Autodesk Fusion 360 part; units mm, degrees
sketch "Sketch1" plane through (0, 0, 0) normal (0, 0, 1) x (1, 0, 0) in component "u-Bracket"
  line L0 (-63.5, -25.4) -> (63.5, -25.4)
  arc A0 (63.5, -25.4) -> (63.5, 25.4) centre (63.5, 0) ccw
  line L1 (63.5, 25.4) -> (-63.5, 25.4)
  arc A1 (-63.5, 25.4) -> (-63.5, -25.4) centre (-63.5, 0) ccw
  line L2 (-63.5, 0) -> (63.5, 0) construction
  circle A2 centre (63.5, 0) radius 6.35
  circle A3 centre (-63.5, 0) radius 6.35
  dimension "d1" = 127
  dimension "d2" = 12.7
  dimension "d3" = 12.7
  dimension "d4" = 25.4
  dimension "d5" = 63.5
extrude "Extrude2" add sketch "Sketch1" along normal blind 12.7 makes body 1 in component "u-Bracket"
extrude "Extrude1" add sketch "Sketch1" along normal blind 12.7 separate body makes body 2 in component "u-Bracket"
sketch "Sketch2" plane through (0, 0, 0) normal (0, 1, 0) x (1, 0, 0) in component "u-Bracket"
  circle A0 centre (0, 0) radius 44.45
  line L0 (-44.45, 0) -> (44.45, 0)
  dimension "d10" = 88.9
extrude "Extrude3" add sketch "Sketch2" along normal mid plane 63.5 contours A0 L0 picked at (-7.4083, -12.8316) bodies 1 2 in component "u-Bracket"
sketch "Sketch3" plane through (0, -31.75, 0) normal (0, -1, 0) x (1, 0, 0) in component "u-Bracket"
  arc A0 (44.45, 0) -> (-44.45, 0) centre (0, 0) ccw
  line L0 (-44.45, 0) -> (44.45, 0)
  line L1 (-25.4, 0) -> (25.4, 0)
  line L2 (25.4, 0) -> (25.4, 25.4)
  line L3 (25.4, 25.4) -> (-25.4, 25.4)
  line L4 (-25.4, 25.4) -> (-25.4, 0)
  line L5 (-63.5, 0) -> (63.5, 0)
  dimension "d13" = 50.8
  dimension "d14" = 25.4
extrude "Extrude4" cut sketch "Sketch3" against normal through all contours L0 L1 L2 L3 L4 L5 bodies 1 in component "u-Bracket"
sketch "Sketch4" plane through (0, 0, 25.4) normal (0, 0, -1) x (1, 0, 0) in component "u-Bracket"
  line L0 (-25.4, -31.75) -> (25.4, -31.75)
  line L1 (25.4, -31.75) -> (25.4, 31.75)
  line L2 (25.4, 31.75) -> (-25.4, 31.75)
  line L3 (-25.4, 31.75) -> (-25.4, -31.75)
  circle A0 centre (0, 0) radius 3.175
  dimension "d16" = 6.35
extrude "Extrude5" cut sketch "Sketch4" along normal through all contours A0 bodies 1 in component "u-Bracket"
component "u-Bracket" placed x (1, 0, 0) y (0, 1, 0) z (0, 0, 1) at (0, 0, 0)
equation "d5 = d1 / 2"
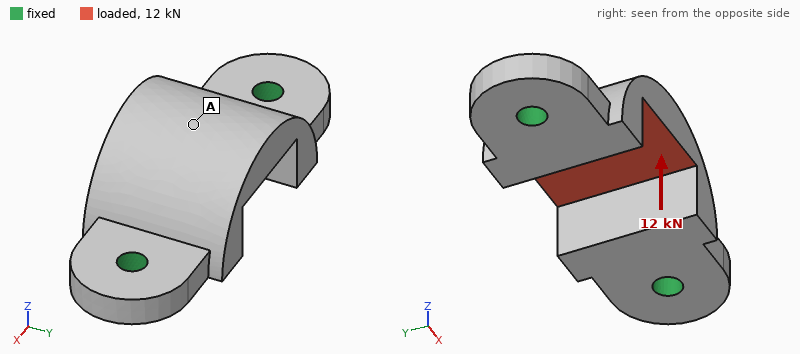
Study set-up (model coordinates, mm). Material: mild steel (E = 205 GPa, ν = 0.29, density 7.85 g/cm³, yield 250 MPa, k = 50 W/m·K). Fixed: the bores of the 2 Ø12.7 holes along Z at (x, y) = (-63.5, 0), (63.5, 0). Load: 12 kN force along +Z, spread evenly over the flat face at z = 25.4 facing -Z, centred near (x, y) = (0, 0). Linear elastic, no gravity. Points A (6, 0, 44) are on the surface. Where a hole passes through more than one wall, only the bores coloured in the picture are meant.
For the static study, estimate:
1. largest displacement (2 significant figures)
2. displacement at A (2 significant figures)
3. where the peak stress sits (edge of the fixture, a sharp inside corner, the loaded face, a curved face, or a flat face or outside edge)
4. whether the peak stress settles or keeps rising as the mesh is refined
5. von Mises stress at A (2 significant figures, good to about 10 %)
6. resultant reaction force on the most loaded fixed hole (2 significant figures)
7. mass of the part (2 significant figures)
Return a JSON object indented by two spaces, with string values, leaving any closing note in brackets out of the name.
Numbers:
{
  "largest displacement": "15 µm",
  "displacement at A": "14 µm",
  "where the peak stress sits": "edge of the fixture",
  "whether the peak stress settles or keeps rising as the mesh is refined": "keeps rising",
  "von Mises stress at A": "14 MPa",
  "resultant reaction force on the most loaded fixed hole": "8.6 kN",
  "mass of the part": "1.3 kg"
}
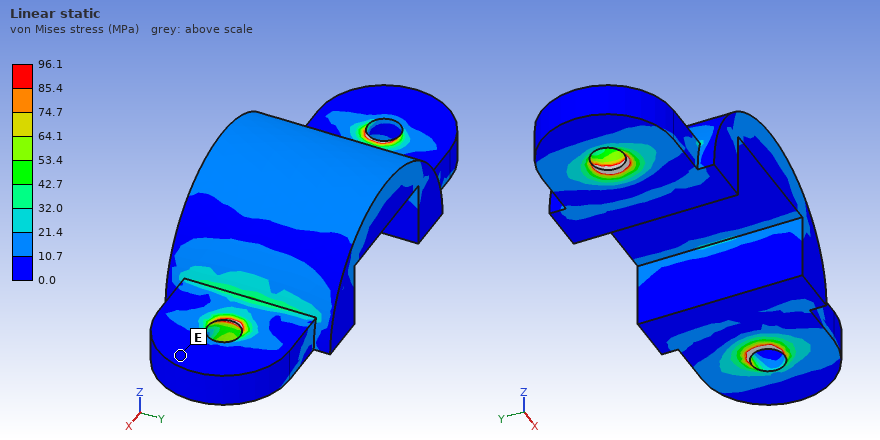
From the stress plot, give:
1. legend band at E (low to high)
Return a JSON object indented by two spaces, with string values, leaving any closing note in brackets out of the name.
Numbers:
{
  "legend band at E": "0.0 to 10.7 MPa"
}
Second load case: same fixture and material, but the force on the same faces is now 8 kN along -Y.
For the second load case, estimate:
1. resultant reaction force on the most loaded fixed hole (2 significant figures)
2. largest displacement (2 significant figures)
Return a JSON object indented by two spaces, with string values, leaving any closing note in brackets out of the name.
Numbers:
{
  "resultant reaction force on the most loaded fixed hole": "4.0 kN",
  "largest displacement": "42 µm"
}
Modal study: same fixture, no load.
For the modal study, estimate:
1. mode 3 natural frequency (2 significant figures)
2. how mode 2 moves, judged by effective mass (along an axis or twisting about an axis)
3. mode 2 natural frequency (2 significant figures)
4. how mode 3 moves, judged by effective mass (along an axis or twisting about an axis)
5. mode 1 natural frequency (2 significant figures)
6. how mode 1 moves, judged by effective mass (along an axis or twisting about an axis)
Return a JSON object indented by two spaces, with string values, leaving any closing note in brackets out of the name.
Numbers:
{
  "mode 3 natural frequency": "5700 Hz",
  "how mode 2 moves, judged by effective mass": "along Z",
  "mode 2 natural frequency": "5300 Hz",
  "how mode 3 moves, judged by effective mass": "along X",
  "mode 1 natural frequency": "2700 Hz",
  "how mode 1 moves, judged by effective mass": "along Y"
}
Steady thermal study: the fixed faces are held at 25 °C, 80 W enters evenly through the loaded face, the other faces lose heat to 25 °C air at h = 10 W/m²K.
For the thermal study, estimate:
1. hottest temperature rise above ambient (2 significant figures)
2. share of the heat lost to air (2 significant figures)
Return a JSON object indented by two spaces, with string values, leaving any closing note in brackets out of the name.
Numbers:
{
  "hottest temperature rise above ambient": "65 K",
  "share of the heat lost to air": "10 %"
}
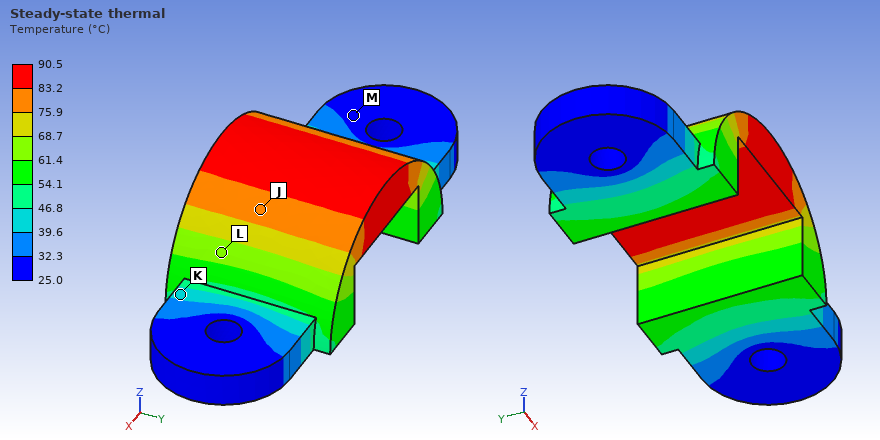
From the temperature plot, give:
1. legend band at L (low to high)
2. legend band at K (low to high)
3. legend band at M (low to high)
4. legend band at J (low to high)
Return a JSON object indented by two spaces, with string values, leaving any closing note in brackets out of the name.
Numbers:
{
  "legend band at L": "61.4 to 68.7 °C",
  "legend band at K": "39.6 to 46.8 °C",
  "legend band at M": "25.0 to 32.3 °C",
  "legend band at J": "75.9 to 83.2 °C"
}
